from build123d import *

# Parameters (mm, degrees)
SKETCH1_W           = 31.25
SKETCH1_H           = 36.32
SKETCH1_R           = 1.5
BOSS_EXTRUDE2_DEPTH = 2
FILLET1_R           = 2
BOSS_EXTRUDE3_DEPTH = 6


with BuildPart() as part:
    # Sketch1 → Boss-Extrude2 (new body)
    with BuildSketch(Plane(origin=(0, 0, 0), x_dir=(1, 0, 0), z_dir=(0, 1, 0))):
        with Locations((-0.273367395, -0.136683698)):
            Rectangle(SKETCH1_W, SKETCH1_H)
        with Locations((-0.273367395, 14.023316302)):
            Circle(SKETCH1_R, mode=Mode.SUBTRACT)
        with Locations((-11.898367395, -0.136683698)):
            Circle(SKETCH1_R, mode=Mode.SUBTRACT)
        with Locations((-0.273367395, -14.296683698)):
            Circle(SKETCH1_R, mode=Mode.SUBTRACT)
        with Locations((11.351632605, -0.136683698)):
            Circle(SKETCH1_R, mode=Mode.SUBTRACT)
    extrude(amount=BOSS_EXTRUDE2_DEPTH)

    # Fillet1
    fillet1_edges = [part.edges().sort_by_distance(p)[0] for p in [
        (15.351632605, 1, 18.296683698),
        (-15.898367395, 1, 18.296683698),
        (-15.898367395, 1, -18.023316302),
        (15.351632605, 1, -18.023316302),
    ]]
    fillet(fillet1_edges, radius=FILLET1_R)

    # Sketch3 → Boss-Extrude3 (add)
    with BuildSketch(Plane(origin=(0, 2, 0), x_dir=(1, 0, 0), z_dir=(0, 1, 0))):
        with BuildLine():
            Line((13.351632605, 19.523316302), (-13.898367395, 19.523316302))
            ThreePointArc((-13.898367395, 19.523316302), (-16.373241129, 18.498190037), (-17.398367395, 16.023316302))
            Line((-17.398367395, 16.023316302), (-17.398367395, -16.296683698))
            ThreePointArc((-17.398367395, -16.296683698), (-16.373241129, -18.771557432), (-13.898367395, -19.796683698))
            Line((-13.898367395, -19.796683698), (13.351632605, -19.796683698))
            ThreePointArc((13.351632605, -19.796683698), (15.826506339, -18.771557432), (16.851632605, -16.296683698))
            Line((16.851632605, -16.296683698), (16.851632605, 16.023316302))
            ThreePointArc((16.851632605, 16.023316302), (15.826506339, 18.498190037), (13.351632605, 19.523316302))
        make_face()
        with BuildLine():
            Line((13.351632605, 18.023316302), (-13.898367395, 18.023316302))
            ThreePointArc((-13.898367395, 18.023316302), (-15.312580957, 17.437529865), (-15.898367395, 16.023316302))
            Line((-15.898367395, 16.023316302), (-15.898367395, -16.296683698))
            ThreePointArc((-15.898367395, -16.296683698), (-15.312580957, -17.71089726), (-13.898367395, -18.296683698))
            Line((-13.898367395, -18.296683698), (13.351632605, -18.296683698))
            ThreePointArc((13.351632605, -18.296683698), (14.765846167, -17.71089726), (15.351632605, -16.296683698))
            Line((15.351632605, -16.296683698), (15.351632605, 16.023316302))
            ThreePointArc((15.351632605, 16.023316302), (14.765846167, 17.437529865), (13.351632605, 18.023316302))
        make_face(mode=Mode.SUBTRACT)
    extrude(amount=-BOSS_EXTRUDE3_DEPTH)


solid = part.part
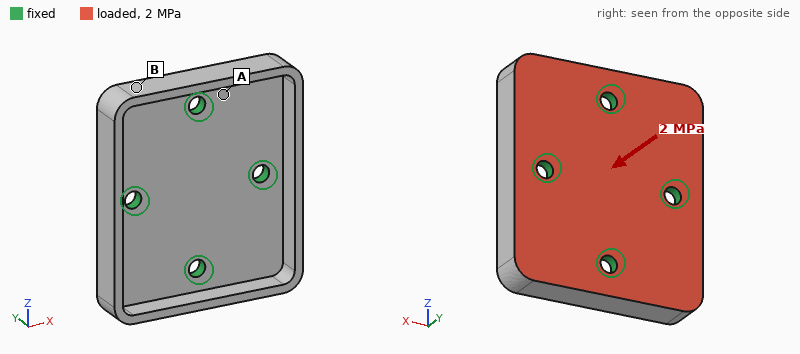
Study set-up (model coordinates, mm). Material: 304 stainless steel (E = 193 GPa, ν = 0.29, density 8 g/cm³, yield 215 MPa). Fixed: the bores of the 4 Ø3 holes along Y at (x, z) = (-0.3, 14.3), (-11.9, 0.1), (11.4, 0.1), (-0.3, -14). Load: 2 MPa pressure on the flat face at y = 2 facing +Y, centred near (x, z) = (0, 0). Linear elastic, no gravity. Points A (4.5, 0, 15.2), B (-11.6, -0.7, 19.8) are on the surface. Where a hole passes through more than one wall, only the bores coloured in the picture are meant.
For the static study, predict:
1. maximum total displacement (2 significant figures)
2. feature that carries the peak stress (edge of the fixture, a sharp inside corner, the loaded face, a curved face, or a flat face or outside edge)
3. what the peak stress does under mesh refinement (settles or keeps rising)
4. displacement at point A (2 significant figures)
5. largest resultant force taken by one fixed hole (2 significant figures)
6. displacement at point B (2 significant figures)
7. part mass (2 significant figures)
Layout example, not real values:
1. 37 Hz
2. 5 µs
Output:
1. 12 µm
2. edge of the fixture
3. keeps rising
4. 3.2 µm
5. 660 N
6. 9.4 µm
7. 27 g
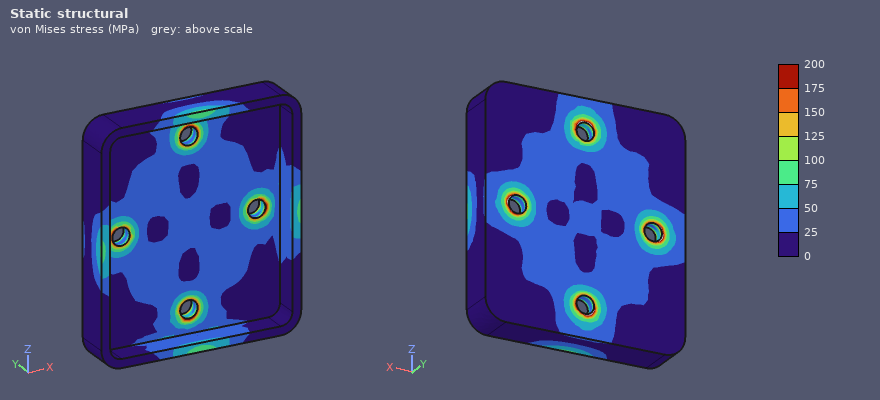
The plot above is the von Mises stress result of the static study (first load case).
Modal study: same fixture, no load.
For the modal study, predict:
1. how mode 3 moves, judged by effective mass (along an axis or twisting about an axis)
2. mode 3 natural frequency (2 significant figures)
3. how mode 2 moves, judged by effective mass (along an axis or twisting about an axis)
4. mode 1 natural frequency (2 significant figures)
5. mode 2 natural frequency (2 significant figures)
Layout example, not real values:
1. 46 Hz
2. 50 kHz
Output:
1. twisting about X
2. 12 kHz
3. twisting about Z
4. 7800 Hz
5. 11 kHz
